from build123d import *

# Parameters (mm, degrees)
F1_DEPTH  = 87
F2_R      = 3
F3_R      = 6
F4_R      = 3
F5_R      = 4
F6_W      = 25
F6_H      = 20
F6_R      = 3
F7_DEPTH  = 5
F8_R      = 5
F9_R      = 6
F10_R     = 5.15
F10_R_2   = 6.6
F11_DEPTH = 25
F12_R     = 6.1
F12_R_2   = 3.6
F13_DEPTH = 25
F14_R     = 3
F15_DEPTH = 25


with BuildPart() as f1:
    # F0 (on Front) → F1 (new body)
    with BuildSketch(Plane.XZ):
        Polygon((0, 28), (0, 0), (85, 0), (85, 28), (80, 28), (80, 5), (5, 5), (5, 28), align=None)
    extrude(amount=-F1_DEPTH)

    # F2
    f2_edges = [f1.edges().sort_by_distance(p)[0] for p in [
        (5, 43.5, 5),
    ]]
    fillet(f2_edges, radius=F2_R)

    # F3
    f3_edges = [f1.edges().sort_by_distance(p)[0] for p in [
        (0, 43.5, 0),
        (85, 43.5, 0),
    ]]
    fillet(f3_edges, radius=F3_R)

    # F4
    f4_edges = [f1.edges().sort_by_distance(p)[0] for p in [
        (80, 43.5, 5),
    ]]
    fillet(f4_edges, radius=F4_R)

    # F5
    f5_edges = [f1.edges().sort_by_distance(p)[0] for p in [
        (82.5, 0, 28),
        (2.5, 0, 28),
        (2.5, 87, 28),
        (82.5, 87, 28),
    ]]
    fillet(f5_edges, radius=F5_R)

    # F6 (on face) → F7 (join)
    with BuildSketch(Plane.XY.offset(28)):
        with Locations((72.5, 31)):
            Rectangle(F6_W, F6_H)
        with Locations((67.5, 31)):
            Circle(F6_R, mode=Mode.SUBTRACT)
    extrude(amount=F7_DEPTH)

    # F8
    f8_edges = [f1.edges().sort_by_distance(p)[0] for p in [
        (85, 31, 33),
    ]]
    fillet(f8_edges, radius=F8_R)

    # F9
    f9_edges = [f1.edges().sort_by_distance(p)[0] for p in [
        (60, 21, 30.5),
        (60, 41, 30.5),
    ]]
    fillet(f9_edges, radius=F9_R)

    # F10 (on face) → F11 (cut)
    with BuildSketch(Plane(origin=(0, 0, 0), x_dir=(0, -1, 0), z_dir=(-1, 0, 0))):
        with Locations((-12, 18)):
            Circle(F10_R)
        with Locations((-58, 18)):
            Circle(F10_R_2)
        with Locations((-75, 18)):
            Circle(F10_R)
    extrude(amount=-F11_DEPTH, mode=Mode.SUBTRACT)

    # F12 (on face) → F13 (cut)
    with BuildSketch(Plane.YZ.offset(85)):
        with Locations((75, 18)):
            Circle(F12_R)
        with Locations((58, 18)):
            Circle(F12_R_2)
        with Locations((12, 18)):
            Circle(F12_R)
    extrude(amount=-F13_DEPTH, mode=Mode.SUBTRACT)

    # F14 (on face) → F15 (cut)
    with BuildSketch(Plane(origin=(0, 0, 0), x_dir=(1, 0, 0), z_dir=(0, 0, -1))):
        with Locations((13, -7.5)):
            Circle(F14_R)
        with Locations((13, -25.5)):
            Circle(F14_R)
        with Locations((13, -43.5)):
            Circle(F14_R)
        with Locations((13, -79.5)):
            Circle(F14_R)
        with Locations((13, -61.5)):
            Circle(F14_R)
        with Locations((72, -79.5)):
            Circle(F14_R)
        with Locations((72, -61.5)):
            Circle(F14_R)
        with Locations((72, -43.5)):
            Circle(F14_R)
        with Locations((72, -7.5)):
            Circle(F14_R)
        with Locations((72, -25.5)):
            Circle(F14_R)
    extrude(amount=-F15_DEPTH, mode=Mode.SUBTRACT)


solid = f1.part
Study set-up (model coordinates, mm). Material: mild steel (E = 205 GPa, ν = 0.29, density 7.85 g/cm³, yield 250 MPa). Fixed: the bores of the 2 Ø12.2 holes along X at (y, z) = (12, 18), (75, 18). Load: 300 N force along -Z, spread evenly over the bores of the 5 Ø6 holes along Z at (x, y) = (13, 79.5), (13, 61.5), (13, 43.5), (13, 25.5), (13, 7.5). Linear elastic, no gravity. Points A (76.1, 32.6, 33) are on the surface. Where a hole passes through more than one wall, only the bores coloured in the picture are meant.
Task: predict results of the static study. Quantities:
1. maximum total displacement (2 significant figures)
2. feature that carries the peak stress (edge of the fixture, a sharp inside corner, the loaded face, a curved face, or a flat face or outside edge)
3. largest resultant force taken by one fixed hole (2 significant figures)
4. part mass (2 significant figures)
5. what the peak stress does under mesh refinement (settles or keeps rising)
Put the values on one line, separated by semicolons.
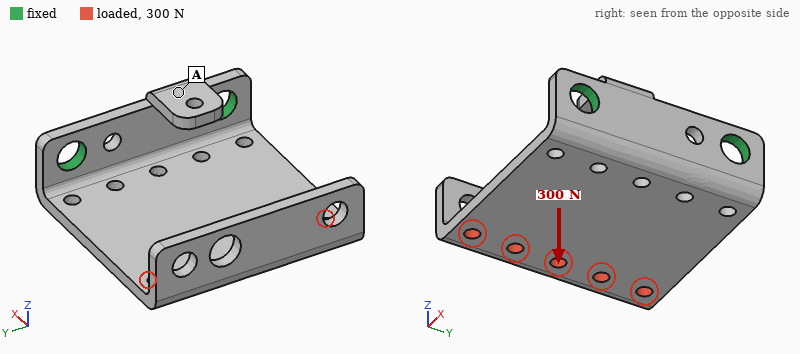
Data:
0.36 mm; edge of the fixture; 160 N; 420 g; keeps rising
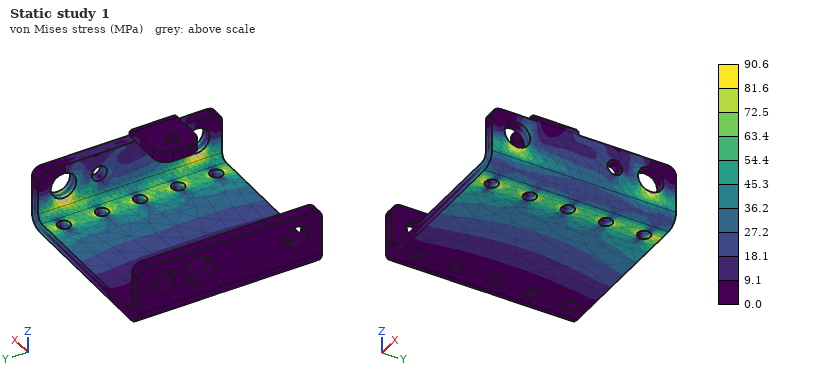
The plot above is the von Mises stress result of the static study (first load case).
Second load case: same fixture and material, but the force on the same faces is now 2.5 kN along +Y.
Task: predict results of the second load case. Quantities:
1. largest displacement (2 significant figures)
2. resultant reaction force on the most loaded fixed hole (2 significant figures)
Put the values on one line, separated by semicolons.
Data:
0.11 mm; 3.0 kN
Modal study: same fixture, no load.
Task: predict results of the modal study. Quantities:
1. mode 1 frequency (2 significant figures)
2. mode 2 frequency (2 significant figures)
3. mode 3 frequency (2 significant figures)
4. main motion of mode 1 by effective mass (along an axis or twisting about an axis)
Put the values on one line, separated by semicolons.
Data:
370 Hz; 980 Hz; 2100 Hz; along Z
